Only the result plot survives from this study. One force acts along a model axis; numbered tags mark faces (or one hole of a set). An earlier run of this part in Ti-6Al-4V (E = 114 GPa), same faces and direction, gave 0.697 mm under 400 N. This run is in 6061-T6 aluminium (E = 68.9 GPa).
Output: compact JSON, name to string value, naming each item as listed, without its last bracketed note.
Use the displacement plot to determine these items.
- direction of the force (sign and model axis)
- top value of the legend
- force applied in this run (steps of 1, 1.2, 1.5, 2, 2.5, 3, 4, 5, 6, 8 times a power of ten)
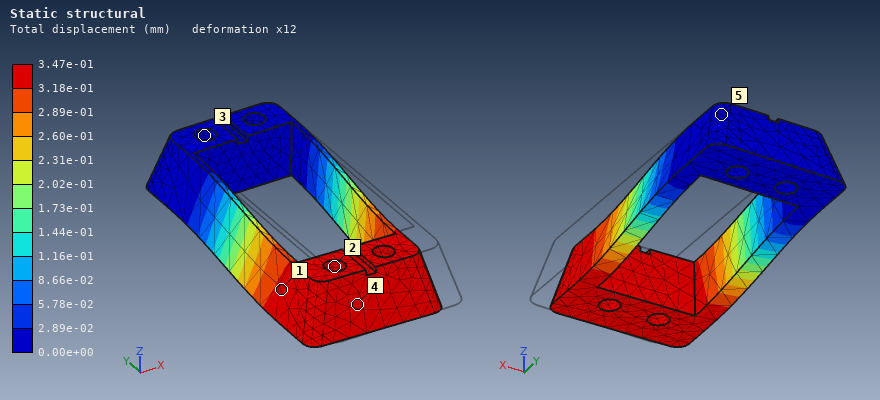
{"direction of the force": "-X", "top value of the legend": "3.47e-01 mm", "force applied in this run": "120 N"}
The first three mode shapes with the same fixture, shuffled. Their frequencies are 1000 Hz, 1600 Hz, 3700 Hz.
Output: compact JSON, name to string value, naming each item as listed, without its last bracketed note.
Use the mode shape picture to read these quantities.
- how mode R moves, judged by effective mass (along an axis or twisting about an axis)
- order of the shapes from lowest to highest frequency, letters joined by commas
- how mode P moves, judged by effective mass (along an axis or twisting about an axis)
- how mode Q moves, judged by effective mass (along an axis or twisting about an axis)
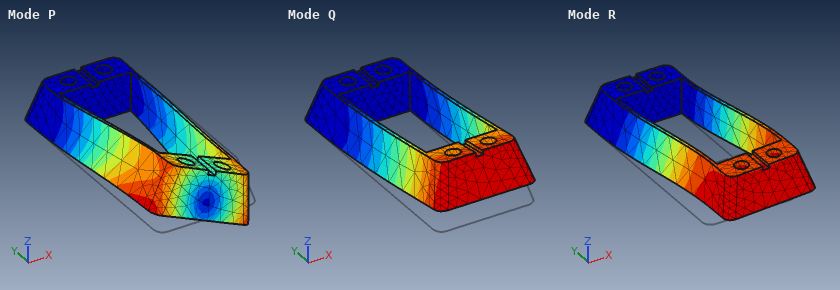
{"how mode R moves, judged by effective mass": "along X", "order of the shapes from lowest to highest frequency, letters joined by commas": "R, Q, P", "how mode P moves, judged by effective mass": "twisting about Y", "how mode Q moves, judged by effective mass": "along Z"}
